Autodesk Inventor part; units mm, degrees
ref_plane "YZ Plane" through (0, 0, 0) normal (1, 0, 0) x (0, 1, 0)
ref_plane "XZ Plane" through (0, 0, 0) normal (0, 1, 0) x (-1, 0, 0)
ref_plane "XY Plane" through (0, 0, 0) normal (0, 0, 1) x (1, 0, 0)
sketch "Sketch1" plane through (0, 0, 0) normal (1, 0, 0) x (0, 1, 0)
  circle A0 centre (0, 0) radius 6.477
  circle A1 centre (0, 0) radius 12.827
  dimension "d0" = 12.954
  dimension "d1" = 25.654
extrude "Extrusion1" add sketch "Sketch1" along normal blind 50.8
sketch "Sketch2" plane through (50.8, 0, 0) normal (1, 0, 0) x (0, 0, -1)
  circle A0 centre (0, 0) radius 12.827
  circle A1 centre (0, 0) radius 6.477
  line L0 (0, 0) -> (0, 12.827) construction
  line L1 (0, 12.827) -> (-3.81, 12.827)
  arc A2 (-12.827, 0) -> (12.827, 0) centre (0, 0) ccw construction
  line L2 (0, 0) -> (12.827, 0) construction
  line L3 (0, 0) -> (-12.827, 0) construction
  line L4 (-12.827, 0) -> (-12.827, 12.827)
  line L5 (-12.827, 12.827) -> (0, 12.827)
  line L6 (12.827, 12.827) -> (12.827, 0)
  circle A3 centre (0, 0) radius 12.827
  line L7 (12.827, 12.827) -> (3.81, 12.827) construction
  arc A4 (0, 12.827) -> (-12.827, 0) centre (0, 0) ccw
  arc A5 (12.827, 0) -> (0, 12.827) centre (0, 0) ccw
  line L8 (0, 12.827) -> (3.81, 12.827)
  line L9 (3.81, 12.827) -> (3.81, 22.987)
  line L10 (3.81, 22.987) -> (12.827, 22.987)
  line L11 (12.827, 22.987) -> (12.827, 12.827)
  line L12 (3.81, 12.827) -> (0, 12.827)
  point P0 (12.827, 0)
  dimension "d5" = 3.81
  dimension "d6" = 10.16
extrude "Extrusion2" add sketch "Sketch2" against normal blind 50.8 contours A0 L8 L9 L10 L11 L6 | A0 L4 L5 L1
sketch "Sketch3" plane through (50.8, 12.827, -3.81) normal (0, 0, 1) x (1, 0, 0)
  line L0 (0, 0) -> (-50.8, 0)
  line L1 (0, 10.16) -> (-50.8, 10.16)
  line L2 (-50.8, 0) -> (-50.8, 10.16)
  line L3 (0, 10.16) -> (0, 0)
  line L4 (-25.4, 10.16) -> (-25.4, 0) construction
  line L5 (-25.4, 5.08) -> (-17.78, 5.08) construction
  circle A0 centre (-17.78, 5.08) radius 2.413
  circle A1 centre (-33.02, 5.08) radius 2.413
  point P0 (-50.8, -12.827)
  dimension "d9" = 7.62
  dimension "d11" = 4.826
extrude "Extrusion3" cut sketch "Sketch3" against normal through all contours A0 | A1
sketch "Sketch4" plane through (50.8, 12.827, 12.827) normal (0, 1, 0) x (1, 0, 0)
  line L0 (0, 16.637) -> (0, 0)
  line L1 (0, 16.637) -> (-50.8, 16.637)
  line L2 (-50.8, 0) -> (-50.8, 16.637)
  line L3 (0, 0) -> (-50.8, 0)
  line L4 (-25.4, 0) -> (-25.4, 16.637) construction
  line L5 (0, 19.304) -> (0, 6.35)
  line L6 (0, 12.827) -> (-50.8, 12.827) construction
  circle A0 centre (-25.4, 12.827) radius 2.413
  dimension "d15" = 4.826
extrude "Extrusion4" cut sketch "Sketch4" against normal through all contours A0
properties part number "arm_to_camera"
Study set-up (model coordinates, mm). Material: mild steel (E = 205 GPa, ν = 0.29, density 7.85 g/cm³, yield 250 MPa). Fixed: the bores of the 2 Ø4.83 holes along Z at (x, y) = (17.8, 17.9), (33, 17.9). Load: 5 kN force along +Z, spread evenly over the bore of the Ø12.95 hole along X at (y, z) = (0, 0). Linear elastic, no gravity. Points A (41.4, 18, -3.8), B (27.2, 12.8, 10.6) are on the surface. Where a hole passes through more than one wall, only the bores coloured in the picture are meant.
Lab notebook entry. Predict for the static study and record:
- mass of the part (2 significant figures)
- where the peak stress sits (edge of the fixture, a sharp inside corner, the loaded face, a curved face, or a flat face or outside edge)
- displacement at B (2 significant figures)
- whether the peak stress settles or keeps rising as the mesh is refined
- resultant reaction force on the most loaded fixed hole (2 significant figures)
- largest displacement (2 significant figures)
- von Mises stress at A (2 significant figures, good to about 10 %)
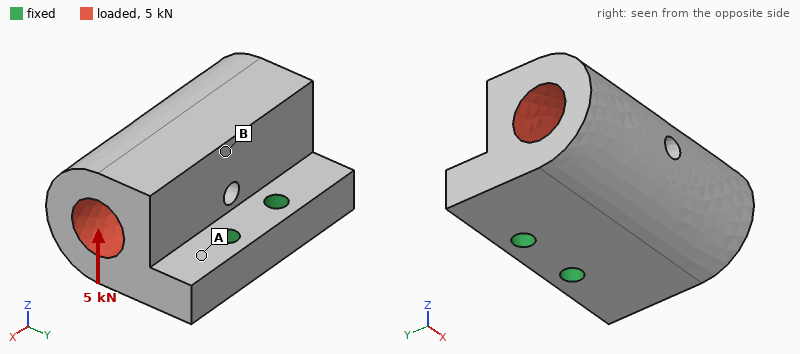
210 g
edge of the fixture
29 µm
keeps rising
2.5 kN
47 µm
54 MPa
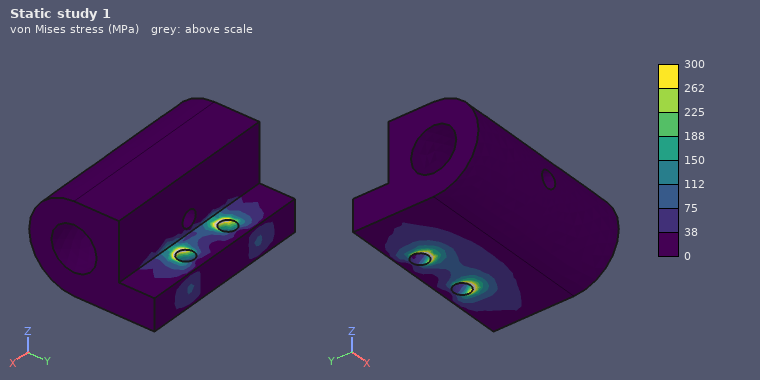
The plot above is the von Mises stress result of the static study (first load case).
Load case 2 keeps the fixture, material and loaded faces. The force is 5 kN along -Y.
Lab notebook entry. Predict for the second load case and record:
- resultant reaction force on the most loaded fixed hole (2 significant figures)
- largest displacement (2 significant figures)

2.5 kN
27 µm
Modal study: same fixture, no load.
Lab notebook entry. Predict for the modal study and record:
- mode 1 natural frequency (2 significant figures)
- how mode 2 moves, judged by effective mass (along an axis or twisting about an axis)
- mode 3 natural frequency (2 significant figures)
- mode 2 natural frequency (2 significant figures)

4300 Hz
along X
9100 Hz
7400 Hz
